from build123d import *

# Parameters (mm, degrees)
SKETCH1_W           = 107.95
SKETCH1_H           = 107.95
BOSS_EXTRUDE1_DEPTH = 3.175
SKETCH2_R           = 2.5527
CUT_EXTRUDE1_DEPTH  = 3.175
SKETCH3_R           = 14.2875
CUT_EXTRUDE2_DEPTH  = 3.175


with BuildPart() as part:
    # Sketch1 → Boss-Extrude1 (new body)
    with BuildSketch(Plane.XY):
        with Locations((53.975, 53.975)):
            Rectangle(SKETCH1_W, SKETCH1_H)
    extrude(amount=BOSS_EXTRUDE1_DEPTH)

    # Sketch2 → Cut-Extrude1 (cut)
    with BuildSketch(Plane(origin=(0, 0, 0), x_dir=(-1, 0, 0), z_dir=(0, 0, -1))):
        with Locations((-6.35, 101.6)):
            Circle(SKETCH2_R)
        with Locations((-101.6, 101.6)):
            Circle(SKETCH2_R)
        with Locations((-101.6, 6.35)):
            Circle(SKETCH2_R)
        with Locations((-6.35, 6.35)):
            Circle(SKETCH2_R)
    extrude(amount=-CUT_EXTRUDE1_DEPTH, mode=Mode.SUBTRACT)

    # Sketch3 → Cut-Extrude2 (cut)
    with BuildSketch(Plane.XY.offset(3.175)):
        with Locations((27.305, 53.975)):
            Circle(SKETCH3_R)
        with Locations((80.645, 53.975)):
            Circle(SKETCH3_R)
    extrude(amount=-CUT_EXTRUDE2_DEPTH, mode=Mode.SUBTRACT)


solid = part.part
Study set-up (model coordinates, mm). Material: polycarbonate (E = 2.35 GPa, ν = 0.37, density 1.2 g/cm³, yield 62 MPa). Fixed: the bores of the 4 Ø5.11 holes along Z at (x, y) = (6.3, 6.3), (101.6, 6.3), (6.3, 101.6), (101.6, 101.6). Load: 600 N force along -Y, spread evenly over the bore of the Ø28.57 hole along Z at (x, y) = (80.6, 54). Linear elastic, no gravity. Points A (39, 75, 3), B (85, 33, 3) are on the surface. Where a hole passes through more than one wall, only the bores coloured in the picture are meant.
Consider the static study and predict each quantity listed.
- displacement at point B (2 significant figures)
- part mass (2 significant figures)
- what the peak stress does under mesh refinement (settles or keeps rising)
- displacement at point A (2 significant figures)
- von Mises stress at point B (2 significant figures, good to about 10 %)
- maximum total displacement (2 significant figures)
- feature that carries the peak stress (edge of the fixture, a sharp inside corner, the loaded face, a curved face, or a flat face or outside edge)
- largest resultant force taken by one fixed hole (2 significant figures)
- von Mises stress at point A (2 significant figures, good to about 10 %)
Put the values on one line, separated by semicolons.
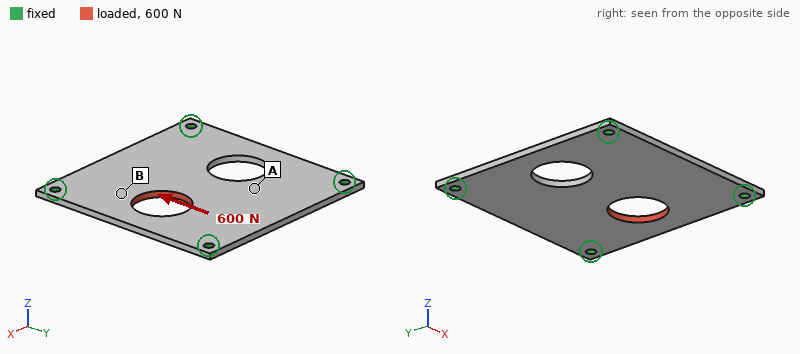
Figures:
56 µm; 39 g; keeps rising; 42 µm; 2.3 MPa; 74 µm; edge of the fixture; 230 N; 1.1 MPa
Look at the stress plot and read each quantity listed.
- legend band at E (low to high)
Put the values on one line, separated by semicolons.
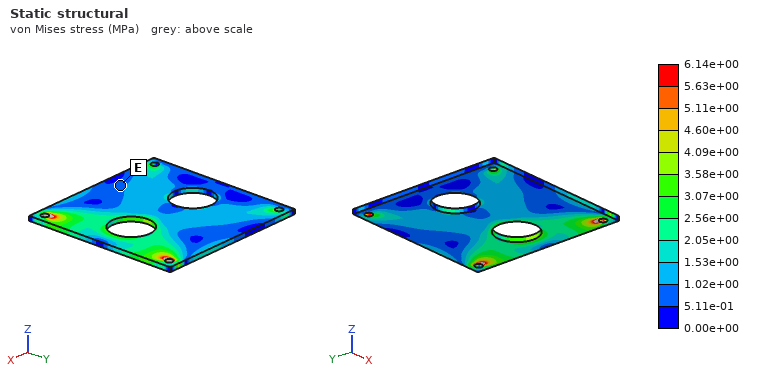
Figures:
5.11e-01 to 1.02e+00 MPa
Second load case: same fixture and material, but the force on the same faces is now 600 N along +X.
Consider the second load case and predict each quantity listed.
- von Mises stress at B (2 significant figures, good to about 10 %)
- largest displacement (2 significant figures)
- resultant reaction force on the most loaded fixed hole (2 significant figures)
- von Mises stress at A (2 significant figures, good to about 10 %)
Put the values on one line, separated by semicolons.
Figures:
3.0 MPa; 0.13 mm; 170 N; 1.5 MPa
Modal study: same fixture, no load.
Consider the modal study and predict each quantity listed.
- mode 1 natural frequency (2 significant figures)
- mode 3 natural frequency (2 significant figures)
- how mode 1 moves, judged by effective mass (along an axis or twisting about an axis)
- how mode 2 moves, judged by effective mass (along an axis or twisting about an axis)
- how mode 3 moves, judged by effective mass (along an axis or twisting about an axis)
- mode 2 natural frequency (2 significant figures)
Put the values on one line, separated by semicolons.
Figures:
330 Hz; 590 Hz; along Z; twisting about X; twisting about Y; 550 Hz
